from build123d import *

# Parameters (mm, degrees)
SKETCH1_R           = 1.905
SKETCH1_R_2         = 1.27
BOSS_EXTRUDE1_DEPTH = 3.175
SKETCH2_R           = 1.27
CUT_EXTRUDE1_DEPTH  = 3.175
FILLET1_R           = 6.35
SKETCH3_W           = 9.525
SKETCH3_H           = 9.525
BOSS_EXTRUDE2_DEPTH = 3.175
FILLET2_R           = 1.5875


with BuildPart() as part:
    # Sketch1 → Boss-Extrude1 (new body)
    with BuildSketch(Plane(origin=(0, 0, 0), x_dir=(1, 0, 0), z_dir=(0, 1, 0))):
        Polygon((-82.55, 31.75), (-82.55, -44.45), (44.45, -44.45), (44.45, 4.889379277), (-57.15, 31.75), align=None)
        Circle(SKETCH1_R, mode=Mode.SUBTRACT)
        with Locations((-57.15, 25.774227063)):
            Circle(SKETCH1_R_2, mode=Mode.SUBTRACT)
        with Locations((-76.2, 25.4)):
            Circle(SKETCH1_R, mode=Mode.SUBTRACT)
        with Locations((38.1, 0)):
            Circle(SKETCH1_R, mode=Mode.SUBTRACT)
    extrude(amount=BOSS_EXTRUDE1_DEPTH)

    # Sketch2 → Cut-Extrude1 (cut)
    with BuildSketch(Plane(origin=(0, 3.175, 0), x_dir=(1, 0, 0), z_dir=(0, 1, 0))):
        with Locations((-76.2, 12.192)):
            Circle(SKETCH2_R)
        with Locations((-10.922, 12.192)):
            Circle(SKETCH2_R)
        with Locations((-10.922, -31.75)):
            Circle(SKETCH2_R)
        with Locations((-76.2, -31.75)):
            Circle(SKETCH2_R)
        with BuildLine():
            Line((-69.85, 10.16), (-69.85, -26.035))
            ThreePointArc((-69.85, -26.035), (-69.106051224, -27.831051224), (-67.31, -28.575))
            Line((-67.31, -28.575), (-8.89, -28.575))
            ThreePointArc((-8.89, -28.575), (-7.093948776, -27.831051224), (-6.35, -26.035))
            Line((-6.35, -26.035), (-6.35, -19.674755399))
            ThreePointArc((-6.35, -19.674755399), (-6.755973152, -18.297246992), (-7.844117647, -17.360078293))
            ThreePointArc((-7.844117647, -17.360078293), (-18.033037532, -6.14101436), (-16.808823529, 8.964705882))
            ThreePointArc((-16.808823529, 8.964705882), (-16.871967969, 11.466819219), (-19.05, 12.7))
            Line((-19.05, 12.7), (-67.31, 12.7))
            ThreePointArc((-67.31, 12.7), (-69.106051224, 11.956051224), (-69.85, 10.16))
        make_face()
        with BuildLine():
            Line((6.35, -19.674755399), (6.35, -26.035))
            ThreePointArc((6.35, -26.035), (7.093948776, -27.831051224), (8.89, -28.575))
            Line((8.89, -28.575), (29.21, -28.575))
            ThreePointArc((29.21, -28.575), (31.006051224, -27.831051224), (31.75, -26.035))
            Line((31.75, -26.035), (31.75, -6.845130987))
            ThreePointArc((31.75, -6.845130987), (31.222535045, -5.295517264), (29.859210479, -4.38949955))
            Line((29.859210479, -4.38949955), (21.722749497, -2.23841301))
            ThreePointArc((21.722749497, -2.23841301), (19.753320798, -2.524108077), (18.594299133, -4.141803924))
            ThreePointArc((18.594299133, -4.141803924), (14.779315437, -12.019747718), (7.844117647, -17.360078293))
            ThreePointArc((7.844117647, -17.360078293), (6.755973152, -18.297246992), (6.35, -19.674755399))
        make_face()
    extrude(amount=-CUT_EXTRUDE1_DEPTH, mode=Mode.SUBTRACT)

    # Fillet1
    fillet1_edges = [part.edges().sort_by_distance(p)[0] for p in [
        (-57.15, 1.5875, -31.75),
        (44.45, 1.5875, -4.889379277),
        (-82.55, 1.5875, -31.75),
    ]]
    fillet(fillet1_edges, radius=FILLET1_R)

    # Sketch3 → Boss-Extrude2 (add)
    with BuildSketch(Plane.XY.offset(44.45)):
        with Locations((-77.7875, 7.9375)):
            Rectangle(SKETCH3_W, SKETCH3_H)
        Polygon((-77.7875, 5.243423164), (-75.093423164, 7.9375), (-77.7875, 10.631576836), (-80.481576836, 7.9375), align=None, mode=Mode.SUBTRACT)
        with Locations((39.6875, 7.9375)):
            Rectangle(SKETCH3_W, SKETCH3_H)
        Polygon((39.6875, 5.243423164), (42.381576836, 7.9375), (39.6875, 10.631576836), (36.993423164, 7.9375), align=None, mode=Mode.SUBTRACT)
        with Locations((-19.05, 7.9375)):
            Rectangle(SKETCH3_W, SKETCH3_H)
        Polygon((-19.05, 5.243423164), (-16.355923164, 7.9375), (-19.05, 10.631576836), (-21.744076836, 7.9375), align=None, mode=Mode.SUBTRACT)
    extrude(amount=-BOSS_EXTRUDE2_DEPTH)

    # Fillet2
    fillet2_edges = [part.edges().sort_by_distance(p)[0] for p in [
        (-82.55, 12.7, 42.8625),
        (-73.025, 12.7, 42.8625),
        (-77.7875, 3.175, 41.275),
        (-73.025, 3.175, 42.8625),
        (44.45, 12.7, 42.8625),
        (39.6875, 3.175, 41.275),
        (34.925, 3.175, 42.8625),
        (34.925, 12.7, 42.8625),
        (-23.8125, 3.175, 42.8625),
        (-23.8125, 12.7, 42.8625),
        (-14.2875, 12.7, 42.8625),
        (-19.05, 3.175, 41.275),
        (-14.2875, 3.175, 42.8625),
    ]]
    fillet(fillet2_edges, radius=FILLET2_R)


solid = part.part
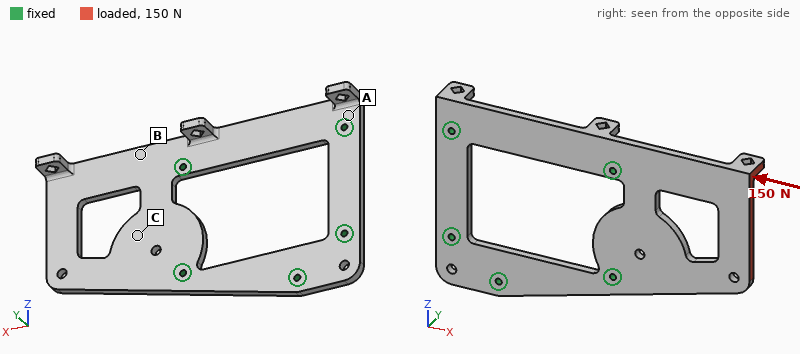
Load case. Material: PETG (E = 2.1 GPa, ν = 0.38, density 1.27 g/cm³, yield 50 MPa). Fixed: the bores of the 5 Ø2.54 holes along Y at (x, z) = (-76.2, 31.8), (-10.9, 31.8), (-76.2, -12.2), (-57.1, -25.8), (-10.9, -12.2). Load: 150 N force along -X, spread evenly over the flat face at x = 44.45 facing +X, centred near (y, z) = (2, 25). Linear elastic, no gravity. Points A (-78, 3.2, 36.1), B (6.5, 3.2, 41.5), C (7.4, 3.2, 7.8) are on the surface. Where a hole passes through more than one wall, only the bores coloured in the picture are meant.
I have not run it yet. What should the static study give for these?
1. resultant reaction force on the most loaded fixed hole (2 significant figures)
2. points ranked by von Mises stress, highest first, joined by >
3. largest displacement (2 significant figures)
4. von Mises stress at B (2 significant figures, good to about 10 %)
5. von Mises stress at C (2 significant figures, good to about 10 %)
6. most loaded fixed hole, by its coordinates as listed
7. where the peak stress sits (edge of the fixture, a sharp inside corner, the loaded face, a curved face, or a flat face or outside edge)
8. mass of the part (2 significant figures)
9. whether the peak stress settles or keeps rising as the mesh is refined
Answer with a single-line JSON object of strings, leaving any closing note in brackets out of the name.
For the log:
{"resultant reaction force on the most loaded fixed hole": "100 N", "points ranked by von Mises stress, highest first, joined by >": "B > C > A", "largest displacement": "1.4 mm", "von Mises stress at B": "4.6 MPa", "von Mises stress at C": "1.2 MPa", "most loaded fixed hole, by its coordinates as listed": "(-10.9, 31.8)", "where the peak stress sits": "edge of the fixture", "mass of the part": "23 g", "whether the peak stress settles or keeps rising as the mesh is refined": "keeps rising"}
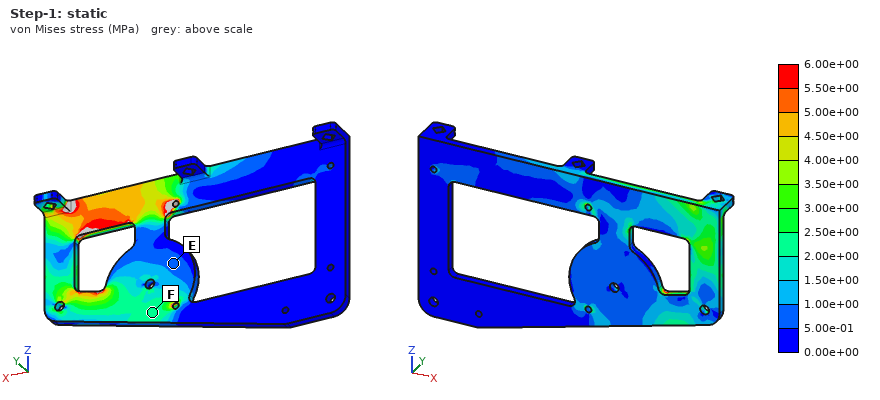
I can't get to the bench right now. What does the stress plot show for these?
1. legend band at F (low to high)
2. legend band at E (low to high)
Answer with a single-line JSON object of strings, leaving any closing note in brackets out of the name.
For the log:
{"legend band at F": "2.00e+00 to 2.50e+00 MPa", "legend band at E": "5.00e-01 to 1.00e+00 MPa"}
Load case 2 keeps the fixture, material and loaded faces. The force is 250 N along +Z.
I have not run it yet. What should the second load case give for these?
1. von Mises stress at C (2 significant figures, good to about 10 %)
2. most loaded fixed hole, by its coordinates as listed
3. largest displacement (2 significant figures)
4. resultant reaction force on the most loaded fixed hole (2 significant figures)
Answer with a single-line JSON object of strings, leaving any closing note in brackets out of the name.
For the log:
{"von Mises stress at C": "4.6 MPa", "most loaded fixed hole, by its coordinates as listed": "(-10.9, -12.2)", "largest displacement": "1.6 mm", "resultant reaction force on the most loaded fixed hole": "310 N"}
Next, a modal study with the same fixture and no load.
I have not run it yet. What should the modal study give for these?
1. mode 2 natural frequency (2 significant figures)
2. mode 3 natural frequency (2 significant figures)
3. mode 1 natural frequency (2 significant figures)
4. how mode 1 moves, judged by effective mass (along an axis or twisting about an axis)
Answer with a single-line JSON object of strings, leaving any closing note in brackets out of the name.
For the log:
{"mode 2 natural frequency": "450 Hz", "mode 3 natural frequency": "890 Hz", "mode 1 natural frequency": "180 Hz", "how mode 1 moves, judged by effective mass": "along Y"}
